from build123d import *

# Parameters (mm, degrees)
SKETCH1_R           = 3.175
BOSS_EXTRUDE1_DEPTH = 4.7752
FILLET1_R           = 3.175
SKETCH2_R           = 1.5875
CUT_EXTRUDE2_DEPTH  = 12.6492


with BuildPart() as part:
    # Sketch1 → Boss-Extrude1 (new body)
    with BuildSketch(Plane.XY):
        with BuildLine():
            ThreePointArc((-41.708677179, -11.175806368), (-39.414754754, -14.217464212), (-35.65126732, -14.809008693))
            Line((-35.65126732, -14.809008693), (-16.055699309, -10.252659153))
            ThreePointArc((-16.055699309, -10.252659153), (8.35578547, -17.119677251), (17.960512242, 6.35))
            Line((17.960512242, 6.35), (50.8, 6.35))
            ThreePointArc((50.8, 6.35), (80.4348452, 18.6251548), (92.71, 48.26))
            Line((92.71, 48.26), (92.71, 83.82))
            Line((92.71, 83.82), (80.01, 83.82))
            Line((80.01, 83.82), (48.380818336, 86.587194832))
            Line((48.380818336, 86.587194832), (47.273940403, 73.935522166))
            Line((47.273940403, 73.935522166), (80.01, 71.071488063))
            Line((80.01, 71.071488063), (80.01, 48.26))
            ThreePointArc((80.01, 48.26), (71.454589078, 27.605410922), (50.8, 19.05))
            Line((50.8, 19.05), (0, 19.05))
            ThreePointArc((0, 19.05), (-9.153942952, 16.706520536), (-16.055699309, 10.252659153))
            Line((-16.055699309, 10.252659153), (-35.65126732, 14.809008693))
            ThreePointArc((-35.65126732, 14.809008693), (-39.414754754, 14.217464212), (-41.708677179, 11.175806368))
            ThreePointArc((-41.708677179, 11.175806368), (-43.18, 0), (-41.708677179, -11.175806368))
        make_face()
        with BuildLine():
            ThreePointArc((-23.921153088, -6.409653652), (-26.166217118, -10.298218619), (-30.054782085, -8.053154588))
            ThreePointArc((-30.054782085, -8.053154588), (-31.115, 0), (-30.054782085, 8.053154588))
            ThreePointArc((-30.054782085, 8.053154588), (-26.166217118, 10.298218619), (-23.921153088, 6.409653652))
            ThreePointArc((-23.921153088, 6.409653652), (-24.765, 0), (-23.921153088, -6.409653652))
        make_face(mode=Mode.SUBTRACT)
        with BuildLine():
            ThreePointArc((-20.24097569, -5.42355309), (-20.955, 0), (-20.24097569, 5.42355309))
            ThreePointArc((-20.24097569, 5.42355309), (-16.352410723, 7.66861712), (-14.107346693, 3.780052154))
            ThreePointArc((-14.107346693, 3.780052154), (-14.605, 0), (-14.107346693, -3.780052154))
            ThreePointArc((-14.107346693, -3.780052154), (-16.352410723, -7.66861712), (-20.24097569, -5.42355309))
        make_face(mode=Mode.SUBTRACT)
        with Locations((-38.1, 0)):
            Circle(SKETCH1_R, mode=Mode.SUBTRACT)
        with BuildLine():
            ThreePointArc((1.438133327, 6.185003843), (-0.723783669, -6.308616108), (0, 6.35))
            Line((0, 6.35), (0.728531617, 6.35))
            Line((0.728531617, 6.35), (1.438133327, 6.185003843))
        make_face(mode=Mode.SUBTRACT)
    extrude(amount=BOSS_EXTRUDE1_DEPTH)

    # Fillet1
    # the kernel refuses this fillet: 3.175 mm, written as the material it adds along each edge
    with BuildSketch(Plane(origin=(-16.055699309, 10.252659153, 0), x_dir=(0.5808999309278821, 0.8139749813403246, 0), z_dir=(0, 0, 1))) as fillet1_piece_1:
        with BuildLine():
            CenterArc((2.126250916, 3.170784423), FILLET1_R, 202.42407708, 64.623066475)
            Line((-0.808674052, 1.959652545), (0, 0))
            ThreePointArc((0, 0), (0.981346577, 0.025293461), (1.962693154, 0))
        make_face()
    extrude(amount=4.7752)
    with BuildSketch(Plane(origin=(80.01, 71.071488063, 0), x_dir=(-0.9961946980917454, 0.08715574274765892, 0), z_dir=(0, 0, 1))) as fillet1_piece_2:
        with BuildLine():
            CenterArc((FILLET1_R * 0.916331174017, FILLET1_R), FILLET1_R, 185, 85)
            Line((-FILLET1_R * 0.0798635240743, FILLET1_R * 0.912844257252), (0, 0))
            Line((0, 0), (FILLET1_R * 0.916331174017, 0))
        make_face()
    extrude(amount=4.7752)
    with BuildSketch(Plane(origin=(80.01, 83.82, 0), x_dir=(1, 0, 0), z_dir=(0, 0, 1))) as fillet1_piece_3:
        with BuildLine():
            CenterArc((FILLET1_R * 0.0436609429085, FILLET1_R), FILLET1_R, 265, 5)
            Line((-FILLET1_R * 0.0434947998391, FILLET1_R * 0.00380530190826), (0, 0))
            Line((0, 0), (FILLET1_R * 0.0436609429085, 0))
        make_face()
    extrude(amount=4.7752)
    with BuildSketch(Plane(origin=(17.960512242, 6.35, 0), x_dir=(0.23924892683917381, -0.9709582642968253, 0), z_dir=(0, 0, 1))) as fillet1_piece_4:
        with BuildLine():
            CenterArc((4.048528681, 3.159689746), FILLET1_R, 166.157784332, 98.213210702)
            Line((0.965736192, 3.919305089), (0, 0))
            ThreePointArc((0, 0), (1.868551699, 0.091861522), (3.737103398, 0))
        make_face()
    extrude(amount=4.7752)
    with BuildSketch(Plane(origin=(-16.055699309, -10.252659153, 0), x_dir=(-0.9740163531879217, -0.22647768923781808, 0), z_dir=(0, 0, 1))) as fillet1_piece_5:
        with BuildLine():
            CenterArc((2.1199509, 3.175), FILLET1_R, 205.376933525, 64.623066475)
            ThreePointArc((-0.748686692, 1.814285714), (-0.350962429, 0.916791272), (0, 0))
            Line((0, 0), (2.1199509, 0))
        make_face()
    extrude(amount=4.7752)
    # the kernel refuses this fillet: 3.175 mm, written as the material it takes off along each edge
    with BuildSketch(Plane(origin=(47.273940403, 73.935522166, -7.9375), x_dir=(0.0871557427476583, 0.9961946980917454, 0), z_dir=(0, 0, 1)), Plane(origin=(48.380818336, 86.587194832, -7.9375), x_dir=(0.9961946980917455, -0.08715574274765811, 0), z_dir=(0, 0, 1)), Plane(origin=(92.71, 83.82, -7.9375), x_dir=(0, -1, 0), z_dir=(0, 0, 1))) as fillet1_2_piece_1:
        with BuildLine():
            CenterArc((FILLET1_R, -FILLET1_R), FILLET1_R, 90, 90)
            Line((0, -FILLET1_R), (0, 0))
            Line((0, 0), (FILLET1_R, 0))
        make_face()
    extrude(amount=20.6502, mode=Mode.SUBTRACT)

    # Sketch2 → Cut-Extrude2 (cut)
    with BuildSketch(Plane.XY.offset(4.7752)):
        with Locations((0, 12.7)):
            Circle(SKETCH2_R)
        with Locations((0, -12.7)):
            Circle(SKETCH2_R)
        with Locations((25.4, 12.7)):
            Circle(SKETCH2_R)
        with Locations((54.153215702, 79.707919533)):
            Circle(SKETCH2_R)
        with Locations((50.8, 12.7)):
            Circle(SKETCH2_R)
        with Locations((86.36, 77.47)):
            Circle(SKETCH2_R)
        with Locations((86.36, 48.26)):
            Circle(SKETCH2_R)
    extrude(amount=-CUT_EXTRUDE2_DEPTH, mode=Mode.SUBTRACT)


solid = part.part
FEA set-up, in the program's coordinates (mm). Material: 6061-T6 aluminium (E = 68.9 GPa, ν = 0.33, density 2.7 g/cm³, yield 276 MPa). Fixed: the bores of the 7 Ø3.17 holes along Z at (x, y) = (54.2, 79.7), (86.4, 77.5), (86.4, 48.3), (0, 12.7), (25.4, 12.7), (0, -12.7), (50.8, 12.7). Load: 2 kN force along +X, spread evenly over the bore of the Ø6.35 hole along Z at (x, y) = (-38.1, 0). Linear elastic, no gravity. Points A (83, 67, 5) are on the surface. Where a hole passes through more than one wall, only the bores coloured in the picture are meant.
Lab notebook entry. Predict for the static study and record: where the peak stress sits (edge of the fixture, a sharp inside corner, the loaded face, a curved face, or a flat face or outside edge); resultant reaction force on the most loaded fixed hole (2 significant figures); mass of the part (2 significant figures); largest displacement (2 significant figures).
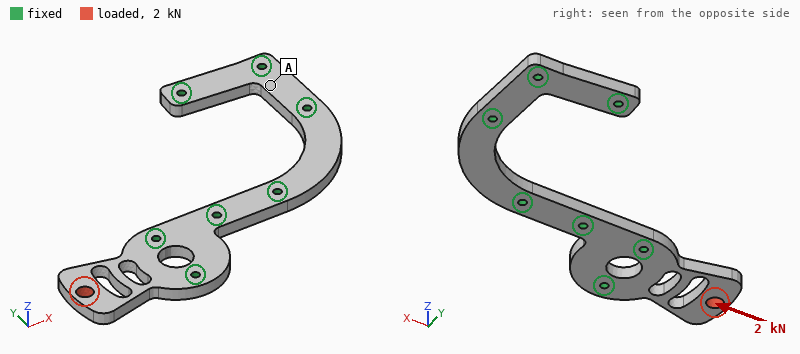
a curved face
1.0 kN
44 g
50 µm
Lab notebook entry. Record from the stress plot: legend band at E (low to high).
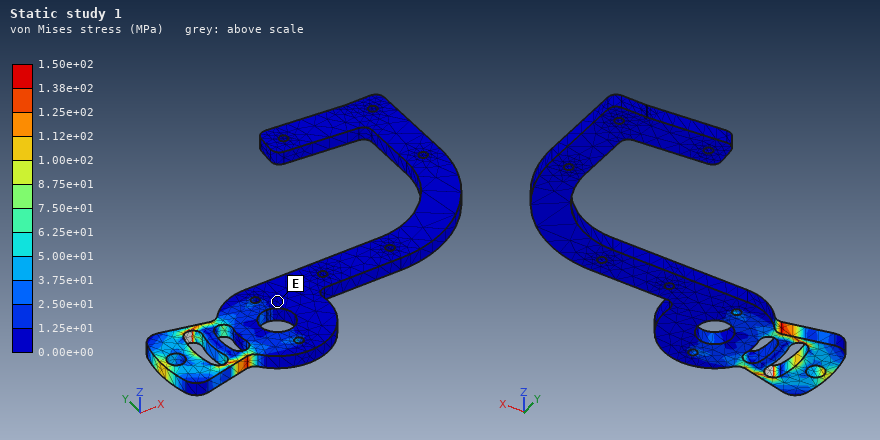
0.00e+00 to 1.25e+01 MPa
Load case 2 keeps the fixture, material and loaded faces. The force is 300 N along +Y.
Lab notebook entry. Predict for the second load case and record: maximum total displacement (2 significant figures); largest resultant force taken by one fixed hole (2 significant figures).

61 µm
440 N
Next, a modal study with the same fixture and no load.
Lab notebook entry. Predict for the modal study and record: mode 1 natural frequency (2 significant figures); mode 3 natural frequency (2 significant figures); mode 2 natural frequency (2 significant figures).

1800 Hz
5800 Hz
5200 Hz
